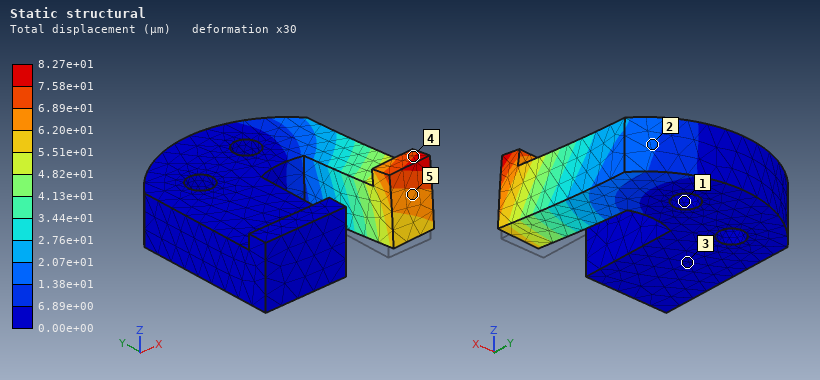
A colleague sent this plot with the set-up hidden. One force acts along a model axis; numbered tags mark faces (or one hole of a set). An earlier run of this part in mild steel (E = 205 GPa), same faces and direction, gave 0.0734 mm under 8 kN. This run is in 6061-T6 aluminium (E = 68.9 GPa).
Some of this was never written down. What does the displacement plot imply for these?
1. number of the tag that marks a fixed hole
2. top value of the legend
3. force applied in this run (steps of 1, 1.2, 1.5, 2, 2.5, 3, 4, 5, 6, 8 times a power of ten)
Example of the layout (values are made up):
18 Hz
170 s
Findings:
1
8.27e+01 µm
3 kN
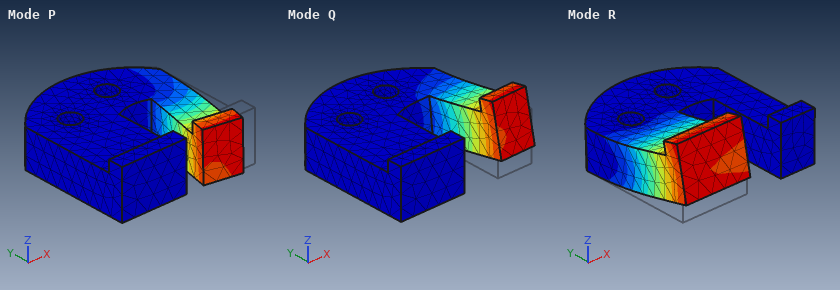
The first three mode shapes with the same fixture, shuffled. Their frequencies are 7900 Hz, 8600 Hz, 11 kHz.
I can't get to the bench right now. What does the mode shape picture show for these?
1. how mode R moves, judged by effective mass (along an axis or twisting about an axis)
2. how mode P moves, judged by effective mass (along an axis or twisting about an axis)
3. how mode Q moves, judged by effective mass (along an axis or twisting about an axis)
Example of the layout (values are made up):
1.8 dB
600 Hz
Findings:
along Z
along X
along Z
